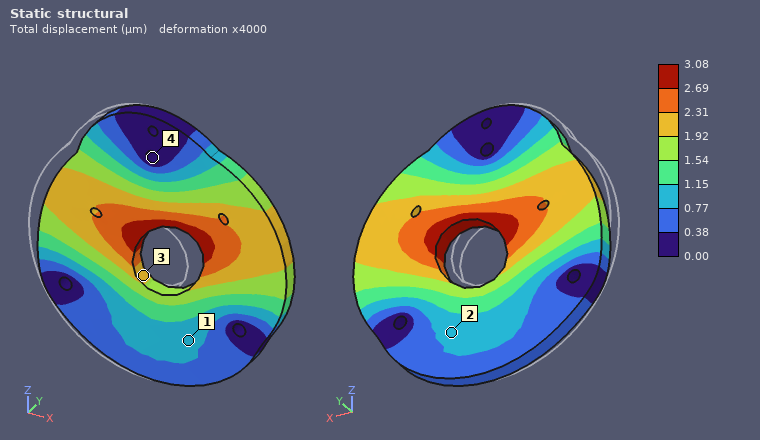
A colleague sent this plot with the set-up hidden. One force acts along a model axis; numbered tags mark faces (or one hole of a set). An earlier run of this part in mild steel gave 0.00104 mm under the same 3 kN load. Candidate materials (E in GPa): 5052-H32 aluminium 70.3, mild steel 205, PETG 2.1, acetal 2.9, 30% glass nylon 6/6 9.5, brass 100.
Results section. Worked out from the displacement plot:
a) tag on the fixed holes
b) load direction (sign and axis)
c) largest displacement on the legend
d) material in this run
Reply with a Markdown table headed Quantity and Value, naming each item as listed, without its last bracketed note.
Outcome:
| Quantity | Value |
|---|---|
| tag on the fixed holes | 4 |
| load direction | +X |
| largest displacement on the legend | 3.08 µm |
| material in this run | 5052-H32 aluminium |
